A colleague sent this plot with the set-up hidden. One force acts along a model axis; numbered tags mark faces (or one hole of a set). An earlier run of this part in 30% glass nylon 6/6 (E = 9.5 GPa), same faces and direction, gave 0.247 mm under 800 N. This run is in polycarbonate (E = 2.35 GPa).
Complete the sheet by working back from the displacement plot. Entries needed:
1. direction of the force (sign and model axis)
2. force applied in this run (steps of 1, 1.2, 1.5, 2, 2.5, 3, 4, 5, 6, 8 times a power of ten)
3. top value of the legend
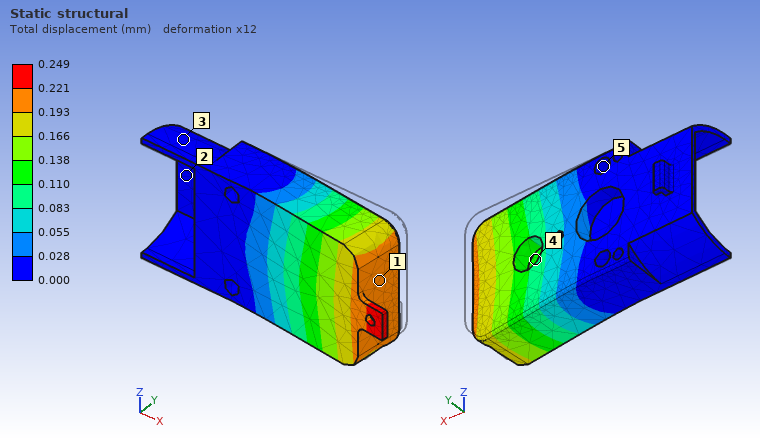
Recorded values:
-Y
200 N
0.249 mm
